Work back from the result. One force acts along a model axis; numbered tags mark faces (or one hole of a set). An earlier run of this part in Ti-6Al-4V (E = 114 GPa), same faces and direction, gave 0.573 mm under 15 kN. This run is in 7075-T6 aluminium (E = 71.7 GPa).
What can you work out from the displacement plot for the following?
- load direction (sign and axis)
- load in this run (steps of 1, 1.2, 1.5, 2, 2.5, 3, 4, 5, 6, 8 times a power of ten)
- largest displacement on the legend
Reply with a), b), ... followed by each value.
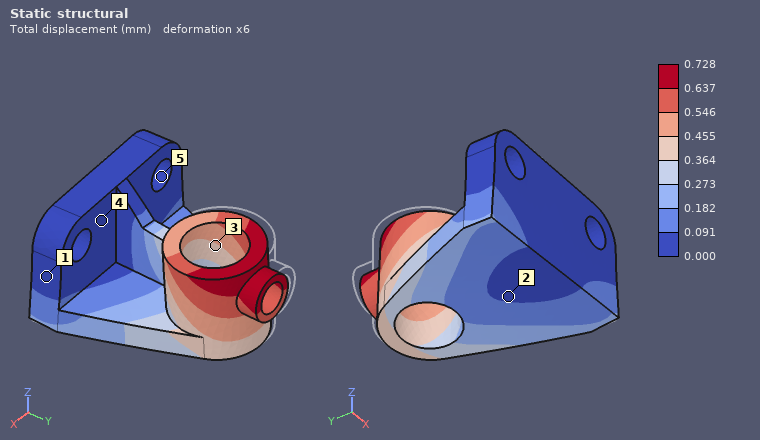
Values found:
a) +X
b) 12 kN
c) 0.728 mm
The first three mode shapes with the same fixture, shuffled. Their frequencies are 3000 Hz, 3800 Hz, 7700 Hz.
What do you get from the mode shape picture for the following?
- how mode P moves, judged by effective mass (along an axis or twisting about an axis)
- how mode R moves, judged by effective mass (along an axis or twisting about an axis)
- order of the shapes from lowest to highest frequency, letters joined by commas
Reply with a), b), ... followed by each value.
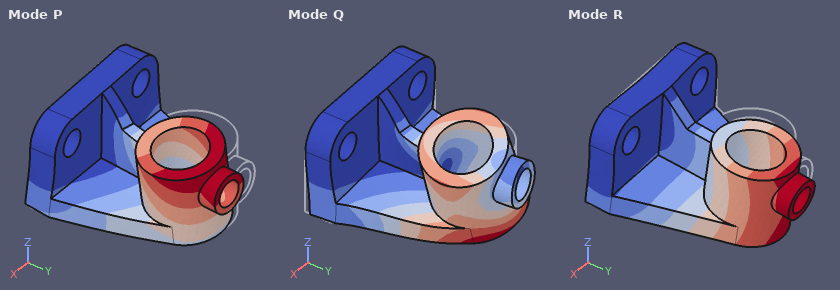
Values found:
a) along X
b) along Z
c) R, P, Q
